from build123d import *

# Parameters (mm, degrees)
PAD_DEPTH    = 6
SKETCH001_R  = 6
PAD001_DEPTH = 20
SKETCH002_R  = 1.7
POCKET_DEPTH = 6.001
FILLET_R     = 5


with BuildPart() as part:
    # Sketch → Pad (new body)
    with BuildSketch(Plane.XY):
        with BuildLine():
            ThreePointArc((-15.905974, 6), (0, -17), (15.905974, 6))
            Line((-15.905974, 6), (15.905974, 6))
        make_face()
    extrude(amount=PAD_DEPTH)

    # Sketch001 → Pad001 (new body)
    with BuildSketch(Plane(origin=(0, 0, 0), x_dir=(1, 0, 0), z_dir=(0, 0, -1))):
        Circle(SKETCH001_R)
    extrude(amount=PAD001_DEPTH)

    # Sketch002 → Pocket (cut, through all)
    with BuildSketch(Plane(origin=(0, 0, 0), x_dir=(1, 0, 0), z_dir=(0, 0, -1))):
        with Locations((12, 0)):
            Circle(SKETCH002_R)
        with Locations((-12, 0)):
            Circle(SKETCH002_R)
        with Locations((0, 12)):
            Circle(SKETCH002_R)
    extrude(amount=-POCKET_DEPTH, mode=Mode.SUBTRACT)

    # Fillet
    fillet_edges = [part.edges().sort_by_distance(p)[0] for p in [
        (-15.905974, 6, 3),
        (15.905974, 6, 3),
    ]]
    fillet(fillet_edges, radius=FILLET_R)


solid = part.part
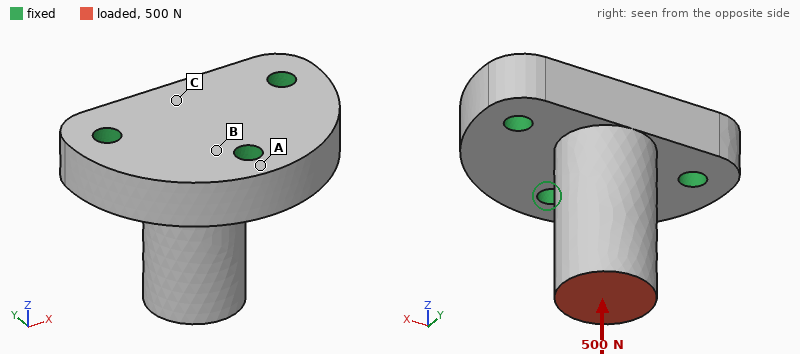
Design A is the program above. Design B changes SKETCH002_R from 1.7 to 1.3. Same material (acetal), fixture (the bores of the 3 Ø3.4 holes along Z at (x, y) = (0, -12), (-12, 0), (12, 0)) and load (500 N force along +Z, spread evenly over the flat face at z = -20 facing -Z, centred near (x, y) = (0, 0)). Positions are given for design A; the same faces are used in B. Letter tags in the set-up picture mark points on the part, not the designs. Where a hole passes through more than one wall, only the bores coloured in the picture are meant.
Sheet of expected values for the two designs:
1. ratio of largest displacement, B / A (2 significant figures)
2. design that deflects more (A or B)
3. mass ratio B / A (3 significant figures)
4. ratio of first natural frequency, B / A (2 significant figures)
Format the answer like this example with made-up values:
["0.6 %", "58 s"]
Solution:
["1.1", "B", "1.01", "0.98"]
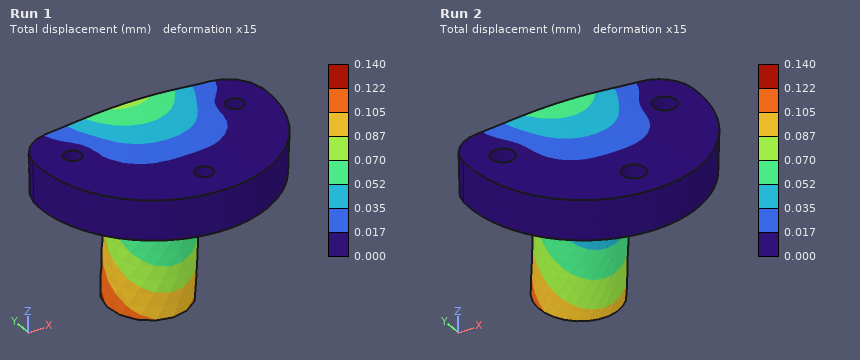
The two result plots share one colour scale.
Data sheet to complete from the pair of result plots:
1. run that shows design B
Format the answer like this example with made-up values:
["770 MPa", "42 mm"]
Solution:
["Run 1"]
